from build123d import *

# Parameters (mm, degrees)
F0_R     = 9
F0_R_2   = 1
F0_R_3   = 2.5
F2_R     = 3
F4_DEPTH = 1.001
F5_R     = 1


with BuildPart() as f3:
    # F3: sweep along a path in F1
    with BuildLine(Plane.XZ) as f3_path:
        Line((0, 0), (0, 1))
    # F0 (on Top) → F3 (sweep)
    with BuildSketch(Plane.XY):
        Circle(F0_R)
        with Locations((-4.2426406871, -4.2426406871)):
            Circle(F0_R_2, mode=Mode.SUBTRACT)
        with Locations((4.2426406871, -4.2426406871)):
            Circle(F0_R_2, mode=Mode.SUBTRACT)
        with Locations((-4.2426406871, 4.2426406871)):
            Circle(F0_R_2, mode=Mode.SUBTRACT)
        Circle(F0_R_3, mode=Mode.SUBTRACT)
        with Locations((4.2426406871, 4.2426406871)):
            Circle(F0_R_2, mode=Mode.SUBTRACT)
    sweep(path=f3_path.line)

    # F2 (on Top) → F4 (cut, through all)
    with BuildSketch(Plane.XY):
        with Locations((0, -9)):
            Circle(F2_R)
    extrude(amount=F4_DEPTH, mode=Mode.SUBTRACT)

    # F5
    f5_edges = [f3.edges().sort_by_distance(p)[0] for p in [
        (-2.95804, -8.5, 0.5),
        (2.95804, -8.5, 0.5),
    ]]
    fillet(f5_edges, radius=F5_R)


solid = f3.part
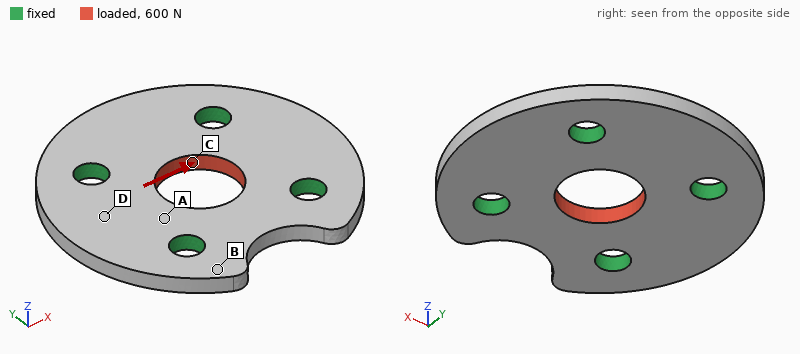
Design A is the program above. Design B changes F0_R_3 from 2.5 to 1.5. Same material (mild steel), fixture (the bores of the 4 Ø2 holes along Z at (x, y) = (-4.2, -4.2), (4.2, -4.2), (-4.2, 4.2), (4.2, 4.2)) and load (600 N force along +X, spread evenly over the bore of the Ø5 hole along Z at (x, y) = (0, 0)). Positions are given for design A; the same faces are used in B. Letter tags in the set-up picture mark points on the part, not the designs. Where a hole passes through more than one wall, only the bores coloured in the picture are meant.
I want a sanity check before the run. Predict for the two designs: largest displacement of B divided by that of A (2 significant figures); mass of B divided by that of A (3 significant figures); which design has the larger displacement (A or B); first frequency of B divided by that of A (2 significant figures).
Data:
1.3
1.06
B
1.0
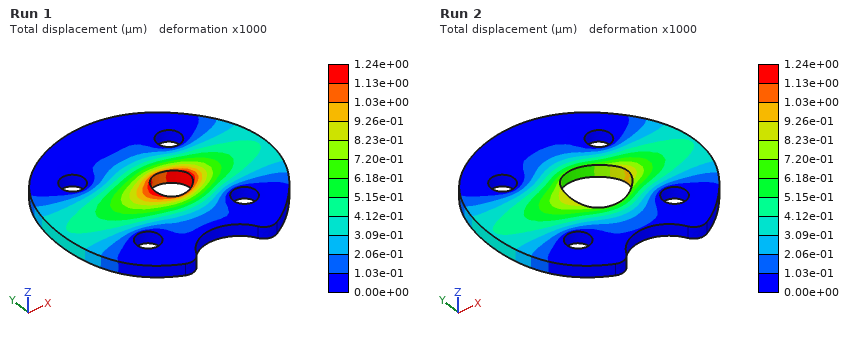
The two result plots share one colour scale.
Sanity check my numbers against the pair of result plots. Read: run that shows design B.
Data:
Run 1
